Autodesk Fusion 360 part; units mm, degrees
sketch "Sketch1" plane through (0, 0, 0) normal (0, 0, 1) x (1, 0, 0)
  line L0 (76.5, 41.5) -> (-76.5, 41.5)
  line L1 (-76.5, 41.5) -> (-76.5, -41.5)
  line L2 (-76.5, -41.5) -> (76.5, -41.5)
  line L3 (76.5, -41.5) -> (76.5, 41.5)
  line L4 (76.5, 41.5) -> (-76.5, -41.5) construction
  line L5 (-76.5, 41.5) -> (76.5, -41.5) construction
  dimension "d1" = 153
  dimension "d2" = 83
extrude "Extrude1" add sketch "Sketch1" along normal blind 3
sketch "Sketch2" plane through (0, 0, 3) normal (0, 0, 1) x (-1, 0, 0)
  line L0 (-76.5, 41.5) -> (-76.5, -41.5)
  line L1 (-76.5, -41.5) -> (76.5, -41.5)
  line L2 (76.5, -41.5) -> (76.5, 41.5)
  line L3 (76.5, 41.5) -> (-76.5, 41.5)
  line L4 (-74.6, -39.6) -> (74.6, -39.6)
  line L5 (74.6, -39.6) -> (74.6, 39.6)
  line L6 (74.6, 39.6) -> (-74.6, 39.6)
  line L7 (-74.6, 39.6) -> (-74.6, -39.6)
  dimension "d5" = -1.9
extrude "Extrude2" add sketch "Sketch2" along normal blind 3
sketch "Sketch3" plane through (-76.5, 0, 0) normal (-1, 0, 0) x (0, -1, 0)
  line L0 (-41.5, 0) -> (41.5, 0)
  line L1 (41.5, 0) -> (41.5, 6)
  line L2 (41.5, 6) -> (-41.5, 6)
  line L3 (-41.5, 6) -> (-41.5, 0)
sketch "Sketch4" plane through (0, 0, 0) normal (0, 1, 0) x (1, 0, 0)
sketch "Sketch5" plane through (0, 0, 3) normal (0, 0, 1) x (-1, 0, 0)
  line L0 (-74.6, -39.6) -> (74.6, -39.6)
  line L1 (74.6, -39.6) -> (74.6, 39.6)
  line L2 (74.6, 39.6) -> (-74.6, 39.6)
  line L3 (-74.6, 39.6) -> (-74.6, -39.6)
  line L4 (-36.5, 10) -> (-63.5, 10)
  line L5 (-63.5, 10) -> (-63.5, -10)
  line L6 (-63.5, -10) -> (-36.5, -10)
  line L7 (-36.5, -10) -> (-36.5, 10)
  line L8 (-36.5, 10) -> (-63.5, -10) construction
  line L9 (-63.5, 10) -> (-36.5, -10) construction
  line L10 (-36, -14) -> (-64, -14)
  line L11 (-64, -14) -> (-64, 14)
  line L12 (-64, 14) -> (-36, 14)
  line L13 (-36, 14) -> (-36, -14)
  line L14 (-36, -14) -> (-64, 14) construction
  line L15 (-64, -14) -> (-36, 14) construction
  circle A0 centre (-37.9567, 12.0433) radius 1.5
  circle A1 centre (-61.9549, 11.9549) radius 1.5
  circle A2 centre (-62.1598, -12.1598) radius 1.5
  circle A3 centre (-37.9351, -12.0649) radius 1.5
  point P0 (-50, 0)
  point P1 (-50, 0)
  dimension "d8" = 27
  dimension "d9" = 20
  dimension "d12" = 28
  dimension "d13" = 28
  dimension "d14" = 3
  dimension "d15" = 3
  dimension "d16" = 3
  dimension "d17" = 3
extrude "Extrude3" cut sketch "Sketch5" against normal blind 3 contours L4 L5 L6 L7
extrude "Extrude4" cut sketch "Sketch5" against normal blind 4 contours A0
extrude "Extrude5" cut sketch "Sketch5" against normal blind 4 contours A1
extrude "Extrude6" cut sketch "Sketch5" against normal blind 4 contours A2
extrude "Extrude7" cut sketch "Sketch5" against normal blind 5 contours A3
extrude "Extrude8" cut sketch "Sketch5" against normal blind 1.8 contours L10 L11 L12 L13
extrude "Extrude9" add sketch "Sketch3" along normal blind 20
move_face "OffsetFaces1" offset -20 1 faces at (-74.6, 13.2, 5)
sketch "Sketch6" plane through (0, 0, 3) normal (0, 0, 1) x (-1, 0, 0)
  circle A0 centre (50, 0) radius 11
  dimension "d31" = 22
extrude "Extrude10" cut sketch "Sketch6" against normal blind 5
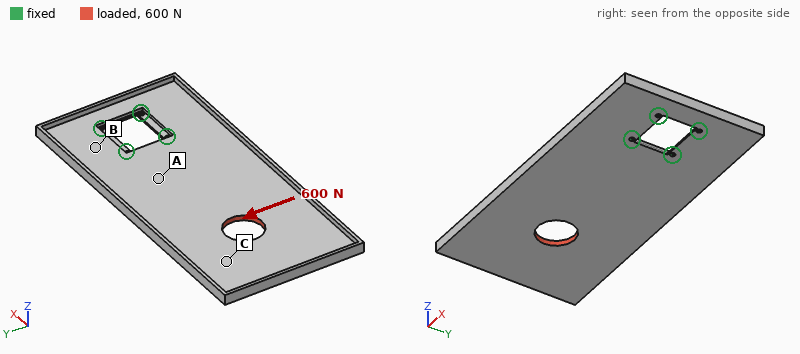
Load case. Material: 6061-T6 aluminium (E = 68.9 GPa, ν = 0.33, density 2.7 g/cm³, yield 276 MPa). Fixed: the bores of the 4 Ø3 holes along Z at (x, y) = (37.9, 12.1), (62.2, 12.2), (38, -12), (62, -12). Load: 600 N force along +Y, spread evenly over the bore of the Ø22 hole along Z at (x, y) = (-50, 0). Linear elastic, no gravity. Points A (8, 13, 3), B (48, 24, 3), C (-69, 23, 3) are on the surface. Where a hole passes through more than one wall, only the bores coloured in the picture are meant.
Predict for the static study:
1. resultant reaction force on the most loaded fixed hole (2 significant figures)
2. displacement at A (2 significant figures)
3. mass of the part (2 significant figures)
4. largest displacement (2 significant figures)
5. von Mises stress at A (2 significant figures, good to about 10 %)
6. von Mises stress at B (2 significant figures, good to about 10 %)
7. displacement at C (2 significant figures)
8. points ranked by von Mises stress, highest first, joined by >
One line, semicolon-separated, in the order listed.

1.0 kN; 21 µm; 120 g; 96 µm; 7.7 MPa; 16 MPa; 74 µm; B > A > C
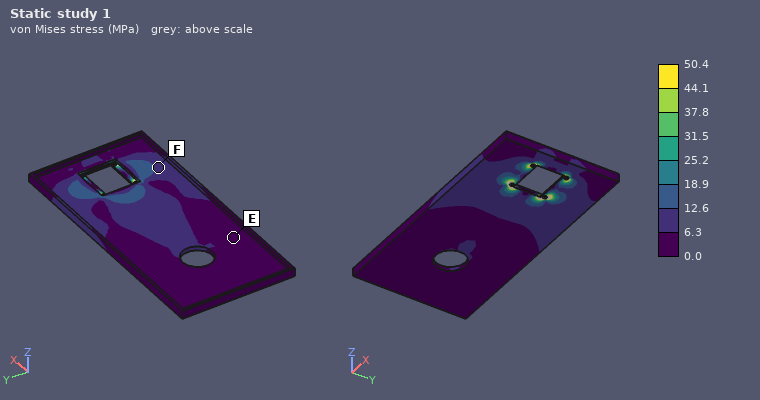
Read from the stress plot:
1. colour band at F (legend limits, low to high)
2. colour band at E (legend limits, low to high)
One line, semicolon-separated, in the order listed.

6.3 to 12.6 MPa; 0.0 to 6.3 MPa
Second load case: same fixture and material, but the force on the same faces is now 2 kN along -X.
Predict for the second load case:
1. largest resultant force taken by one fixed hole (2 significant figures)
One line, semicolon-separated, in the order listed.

730 N
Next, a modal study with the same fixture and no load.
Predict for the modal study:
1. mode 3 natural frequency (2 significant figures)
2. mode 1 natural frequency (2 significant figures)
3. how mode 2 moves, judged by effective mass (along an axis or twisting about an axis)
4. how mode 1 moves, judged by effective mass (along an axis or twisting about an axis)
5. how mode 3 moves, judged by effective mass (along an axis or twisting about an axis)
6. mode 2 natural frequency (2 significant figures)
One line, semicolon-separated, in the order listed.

820 Hz; 140 Hz; twisting about X; along Z; along Z; 410 Hz
